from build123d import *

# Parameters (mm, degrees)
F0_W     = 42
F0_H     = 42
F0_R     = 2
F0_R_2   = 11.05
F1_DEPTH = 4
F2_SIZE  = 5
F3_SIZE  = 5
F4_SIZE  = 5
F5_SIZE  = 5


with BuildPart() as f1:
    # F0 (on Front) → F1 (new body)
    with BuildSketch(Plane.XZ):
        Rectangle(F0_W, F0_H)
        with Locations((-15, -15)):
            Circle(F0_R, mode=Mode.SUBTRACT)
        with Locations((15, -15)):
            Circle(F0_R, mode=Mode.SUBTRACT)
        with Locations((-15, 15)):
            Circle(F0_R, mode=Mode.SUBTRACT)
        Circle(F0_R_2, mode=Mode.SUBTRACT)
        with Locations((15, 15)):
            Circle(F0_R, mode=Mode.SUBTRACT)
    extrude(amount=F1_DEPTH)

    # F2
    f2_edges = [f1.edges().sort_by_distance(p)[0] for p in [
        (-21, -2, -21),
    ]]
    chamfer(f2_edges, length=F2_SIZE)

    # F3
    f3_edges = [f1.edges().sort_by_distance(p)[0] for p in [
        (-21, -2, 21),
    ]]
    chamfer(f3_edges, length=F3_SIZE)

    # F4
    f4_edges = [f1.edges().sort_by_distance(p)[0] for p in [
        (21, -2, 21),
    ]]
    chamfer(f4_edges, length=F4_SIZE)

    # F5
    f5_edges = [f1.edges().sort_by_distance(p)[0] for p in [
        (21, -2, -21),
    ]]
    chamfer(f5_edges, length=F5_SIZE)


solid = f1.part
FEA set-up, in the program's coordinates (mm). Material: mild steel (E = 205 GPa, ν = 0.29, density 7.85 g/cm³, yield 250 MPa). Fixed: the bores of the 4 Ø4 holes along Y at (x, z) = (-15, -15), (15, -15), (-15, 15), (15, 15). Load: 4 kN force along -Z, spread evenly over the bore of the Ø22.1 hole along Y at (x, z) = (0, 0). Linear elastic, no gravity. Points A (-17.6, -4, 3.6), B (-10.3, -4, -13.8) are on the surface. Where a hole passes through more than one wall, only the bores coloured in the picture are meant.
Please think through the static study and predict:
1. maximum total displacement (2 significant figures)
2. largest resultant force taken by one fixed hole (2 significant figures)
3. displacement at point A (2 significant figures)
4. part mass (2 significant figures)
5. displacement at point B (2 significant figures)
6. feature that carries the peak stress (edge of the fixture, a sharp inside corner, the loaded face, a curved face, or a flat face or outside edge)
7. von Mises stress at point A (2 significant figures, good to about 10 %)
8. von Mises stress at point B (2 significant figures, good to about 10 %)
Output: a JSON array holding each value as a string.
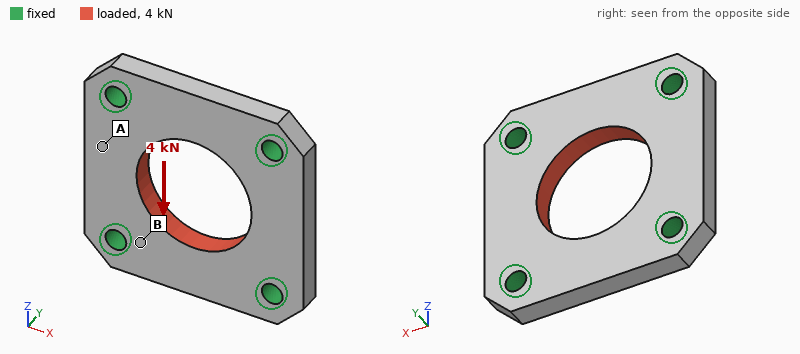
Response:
["2.8 µm", "1.0 kN", "0.59 µm", "40 g", "0.90 µm", "edge of the fixture", "11 MPa", "22 MPa"]
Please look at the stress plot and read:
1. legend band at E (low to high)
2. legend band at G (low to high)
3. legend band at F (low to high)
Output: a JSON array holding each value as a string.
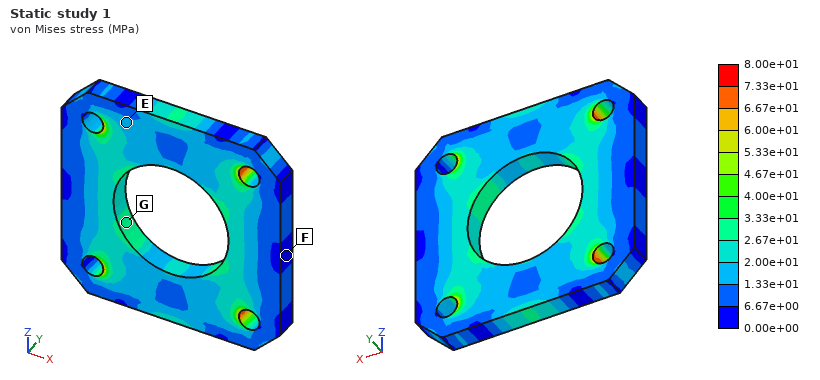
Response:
["1.33e+01 to 2.00e+01 MPa", "2.67e+01 to 3.33e+01 MPa", "0.00e+00 to 6.67e+00 MPa"]
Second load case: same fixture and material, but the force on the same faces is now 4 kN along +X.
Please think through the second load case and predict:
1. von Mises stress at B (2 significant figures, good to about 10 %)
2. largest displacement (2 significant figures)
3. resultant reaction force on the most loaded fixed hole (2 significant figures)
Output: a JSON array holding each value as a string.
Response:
["24 MPa", "2.8 µm", "1.0 kN"]
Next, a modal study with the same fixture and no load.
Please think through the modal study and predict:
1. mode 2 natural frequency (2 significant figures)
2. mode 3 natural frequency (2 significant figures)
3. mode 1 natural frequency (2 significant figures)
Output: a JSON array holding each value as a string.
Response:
["24 kHz", "24 kHz", "24 kHz"]
